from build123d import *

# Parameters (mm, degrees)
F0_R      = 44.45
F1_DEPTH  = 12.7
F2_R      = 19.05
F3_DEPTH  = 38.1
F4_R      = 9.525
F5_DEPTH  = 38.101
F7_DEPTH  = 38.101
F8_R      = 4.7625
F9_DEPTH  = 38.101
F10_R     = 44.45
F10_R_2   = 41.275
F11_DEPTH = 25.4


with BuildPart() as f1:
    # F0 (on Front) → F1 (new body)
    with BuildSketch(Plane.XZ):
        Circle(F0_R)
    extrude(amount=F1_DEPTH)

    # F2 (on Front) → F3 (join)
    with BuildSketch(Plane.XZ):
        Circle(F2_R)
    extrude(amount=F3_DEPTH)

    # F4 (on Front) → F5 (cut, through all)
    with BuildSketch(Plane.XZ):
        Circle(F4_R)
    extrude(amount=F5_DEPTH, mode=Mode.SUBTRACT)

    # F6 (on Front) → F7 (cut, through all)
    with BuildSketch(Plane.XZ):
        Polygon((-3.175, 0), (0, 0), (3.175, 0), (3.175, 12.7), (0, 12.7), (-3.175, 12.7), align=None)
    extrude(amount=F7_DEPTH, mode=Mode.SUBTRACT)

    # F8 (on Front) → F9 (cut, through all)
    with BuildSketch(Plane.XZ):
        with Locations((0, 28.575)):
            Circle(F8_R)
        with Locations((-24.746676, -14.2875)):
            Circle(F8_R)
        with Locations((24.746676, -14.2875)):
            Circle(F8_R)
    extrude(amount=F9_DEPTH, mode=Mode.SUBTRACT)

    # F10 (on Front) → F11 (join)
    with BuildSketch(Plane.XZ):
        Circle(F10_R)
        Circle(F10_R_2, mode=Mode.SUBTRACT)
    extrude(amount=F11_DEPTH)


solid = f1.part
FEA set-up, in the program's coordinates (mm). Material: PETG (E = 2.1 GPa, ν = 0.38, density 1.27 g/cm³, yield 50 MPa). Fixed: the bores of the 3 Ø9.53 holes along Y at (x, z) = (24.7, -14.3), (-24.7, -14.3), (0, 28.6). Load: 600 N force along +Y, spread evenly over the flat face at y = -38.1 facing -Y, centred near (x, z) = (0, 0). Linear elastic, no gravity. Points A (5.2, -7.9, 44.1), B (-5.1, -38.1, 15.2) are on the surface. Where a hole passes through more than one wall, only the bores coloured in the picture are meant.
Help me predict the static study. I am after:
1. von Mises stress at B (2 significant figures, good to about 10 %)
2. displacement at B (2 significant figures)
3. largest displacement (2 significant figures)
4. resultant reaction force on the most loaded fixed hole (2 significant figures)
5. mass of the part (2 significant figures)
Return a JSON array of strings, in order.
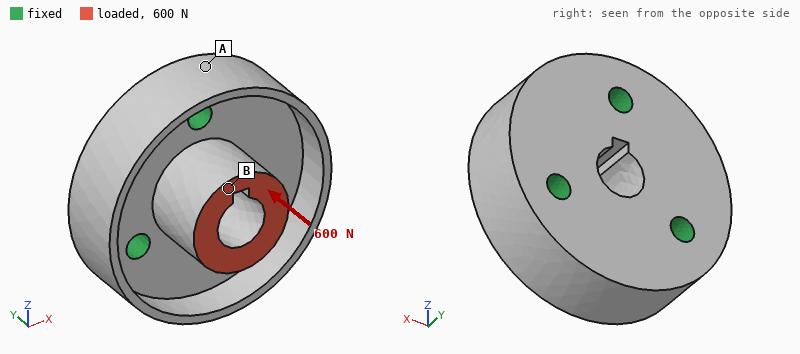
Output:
["0.75 MPa", "21 µm", "22 µm", "210 N", "130 g"]
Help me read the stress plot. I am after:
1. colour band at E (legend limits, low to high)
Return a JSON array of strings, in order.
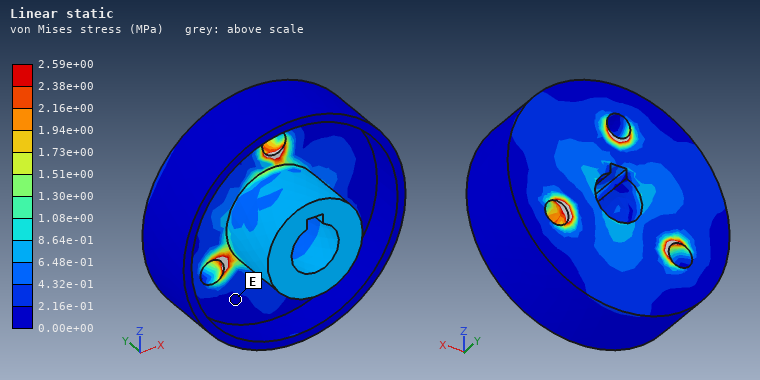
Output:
["0.00e+00 to 2.16e-01 MPa"]
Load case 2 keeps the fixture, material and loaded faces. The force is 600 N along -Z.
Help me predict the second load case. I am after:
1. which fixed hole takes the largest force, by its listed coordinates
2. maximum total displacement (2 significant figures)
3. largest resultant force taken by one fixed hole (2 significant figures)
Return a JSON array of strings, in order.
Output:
["(0, 28.6)", "0.13 mm", "480 N"]
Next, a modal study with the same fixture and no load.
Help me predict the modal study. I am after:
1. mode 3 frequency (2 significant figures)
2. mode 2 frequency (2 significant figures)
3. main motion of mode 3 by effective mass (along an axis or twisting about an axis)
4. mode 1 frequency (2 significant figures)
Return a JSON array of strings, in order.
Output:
["2900 Hz", "2400 Hz", "along Y", "2400 Hz"]
